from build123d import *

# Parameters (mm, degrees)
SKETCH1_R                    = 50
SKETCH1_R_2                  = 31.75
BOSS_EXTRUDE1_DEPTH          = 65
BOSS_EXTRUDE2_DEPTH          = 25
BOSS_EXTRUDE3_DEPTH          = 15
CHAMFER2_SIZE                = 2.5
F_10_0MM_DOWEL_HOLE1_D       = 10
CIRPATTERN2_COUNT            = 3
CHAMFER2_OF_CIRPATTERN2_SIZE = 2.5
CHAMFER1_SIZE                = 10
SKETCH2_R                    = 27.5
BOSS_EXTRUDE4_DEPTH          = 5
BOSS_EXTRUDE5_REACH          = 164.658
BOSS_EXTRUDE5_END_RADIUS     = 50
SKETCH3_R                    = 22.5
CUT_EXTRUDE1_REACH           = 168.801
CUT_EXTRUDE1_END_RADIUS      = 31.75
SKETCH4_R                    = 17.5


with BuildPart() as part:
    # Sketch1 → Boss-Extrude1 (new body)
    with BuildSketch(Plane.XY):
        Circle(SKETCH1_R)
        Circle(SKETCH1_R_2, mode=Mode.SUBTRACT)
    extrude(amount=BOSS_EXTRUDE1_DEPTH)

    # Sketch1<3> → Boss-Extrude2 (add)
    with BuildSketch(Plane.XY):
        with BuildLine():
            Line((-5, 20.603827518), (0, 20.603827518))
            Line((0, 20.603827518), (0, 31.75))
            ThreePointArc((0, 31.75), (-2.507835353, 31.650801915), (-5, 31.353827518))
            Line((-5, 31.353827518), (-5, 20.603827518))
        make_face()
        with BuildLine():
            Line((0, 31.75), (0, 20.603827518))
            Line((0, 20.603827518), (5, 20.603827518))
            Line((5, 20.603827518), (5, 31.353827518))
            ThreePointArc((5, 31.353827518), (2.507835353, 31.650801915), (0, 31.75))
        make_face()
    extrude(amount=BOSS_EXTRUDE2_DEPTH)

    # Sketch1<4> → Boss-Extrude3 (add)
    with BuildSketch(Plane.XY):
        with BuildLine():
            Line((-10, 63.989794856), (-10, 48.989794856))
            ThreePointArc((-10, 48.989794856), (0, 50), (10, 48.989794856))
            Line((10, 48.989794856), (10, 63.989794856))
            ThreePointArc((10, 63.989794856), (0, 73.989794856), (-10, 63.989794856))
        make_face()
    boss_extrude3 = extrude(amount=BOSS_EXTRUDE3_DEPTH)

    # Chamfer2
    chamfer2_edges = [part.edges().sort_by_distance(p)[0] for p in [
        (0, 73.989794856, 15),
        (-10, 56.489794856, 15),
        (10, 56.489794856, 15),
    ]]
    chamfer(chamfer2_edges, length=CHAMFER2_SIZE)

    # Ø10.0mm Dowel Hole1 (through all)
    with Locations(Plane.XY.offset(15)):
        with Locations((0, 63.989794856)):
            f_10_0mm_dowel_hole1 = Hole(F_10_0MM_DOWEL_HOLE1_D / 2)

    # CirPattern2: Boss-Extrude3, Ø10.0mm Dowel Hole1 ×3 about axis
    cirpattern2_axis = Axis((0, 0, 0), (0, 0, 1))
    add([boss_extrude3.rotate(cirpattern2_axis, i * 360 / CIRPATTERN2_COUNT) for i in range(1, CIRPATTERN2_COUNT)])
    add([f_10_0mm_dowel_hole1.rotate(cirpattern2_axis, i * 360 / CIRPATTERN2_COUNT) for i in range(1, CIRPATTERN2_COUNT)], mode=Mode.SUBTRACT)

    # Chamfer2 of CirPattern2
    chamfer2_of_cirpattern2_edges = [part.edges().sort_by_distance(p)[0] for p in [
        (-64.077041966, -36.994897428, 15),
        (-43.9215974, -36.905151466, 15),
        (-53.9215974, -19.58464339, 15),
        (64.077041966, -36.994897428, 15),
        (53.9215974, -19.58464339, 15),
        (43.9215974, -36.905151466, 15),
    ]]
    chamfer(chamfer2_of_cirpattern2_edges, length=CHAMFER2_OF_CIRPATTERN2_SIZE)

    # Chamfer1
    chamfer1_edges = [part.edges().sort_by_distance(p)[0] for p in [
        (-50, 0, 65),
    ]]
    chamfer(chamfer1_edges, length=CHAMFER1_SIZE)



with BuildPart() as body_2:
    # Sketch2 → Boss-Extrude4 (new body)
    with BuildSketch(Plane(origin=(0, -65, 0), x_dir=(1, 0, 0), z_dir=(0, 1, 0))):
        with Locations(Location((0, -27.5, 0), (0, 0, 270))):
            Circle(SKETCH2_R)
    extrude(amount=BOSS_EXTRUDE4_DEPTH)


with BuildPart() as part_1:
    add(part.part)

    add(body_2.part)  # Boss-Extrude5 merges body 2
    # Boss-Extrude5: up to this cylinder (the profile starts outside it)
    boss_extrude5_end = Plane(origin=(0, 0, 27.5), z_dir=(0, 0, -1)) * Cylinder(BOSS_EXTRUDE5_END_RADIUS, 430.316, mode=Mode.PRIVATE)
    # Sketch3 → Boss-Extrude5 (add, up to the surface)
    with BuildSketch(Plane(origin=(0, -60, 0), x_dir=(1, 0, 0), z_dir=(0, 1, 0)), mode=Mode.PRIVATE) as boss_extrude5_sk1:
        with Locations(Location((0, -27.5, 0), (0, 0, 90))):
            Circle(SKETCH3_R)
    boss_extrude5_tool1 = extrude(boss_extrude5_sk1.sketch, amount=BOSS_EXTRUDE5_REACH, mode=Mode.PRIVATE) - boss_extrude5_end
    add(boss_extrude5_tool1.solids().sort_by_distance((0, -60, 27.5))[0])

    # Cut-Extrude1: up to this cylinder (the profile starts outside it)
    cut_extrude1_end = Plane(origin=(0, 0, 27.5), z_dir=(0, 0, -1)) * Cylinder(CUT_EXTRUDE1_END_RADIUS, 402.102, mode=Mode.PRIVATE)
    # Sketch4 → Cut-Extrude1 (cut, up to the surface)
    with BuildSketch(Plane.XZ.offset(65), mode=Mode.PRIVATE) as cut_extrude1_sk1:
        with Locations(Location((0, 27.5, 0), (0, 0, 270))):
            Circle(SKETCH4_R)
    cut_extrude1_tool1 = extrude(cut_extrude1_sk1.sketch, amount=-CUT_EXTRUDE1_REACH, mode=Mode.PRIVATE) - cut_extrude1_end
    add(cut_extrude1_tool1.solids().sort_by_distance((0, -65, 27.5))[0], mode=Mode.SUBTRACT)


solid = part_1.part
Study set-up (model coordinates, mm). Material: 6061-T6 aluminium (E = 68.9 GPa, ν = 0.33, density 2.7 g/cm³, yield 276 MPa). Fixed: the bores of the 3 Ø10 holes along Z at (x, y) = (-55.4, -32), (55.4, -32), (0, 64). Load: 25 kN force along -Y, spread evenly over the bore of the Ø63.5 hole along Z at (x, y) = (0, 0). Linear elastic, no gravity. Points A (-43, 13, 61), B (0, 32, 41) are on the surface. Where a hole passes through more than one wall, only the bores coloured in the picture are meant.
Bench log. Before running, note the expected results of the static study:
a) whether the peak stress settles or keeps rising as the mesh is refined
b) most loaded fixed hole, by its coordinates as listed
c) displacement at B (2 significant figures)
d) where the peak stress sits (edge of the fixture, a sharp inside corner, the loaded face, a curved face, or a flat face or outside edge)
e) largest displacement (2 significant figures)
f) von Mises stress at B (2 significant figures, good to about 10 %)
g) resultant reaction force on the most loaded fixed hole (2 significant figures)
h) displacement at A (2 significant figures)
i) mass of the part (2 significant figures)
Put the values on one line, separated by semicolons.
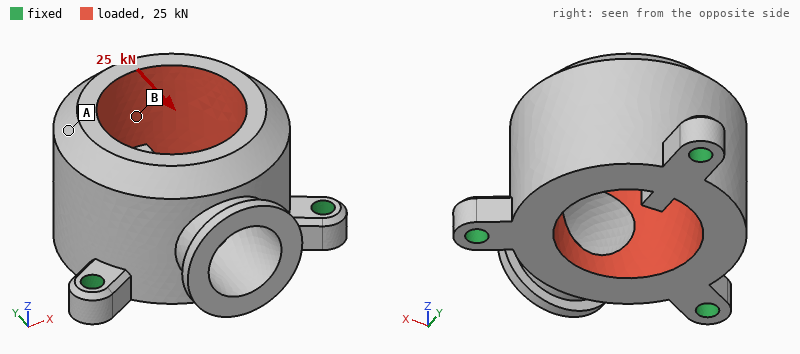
keeps rising; (0, 64); 34 µm; edge of the fixture; 82 µm; 26 MPa; 12 kN; 59 µm; 820 g
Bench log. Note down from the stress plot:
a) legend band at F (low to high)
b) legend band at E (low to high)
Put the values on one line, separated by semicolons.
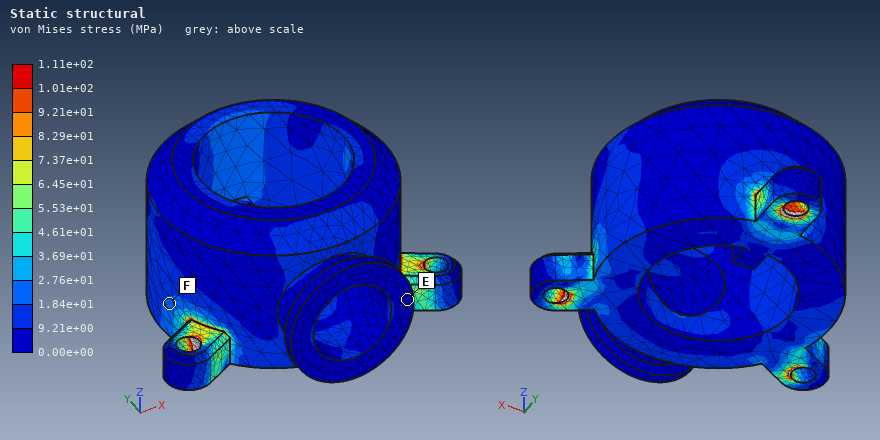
1.84e+01 to 2.76e+01 MPa; 0.00e+00 to 9.21e+00 MPa
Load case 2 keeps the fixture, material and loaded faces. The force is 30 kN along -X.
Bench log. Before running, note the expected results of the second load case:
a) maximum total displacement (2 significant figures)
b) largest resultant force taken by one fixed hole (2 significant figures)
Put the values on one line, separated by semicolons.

0.10 mm; 13 kN
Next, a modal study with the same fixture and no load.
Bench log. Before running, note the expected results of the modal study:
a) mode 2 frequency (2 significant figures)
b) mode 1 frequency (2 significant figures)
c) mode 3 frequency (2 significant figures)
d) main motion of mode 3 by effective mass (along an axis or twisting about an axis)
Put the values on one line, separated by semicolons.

3700 Hz; 3600 Hz; 4700 Hz; along Z
